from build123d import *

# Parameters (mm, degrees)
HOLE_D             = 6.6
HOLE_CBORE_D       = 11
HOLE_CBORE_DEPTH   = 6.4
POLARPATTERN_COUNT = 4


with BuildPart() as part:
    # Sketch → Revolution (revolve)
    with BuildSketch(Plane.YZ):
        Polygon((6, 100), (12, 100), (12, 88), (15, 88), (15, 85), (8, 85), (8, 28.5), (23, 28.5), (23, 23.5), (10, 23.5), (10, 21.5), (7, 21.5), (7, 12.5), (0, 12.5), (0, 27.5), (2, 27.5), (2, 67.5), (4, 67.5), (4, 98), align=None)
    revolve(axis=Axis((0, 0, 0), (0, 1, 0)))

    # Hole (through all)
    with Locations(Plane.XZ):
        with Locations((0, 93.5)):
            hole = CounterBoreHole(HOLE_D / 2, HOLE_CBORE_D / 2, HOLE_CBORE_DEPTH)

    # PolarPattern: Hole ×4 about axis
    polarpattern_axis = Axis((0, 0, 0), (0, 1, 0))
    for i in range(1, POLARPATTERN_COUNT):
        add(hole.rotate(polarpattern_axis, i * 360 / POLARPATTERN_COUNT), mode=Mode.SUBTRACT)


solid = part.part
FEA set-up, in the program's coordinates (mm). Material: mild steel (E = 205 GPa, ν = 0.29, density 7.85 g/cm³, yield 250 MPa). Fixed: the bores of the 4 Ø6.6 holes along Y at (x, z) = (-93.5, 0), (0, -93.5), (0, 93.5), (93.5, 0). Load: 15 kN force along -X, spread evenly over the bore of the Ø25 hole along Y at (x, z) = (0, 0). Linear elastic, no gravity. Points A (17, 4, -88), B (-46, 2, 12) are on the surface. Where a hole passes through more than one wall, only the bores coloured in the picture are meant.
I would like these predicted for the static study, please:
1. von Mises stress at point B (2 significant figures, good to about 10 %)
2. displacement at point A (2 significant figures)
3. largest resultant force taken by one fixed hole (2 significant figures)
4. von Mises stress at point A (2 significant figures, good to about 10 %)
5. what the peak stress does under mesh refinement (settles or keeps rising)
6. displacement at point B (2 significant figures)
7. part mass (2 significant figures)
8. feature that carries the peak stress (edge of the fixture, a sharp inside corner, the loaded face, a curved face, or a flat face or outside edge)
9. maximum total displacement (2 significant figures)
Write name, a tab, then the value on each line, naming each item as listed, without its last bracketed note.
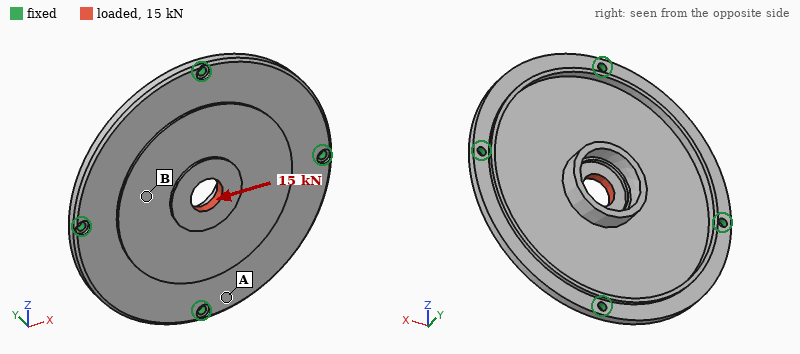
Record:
von Mises stress at point B	20 MPa
displacement at point A	3.5 µm
largest resultant force taken by one fixed hole	4.3 kN
von Mises stress at point A	9.4 MPa
what the peak stress does under mesh refinement	keeps rising
displacement at point B	7.1 µm
part mass	1.6 kg
feature that carries the peak stress	edge of the fixture
maximum total displacement	12 µm
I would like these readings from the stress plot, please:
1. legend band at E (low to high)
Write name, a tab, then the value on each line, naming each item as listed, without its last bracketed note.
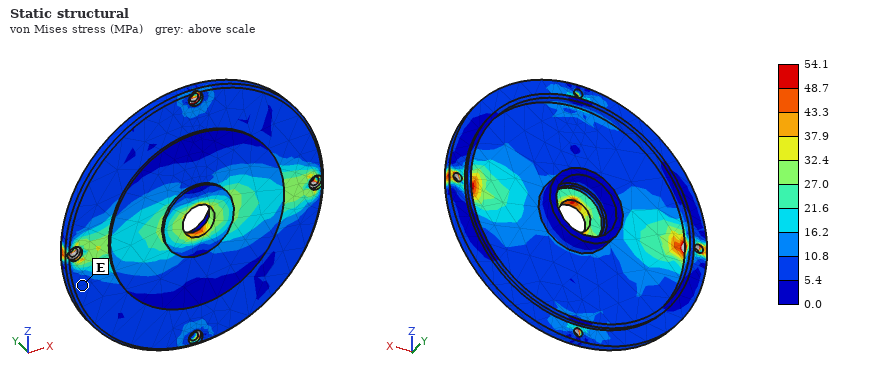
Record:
legend band at E	5.4 to 10.8 MPa
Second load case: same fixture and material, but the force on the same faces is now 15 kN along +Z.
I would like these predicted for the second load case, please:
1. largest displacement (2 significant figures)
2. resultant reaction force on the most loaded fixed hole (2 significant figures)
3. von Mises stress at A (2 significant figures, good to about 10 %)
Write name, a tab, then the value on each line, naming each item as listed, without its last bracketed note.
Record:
largest displacement	12 µm
resultant reaction force on the most loaded fixed hole	4.3 kN
von Mises stress at A	11 MPa
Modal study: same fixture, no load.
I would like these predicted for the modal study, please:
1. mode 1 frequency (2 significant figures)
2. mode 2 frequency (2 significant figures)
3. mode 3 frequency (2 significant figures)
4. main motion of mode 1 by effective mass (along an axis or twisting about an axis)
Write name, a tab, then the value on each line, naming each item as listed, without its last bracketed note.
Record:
mode 1 frequency	1300 Hz
mode 2 frequency	1900 Hz
mode 3 frequency	1900 Hz
main motion of mode 1 by effective mass	along Y
